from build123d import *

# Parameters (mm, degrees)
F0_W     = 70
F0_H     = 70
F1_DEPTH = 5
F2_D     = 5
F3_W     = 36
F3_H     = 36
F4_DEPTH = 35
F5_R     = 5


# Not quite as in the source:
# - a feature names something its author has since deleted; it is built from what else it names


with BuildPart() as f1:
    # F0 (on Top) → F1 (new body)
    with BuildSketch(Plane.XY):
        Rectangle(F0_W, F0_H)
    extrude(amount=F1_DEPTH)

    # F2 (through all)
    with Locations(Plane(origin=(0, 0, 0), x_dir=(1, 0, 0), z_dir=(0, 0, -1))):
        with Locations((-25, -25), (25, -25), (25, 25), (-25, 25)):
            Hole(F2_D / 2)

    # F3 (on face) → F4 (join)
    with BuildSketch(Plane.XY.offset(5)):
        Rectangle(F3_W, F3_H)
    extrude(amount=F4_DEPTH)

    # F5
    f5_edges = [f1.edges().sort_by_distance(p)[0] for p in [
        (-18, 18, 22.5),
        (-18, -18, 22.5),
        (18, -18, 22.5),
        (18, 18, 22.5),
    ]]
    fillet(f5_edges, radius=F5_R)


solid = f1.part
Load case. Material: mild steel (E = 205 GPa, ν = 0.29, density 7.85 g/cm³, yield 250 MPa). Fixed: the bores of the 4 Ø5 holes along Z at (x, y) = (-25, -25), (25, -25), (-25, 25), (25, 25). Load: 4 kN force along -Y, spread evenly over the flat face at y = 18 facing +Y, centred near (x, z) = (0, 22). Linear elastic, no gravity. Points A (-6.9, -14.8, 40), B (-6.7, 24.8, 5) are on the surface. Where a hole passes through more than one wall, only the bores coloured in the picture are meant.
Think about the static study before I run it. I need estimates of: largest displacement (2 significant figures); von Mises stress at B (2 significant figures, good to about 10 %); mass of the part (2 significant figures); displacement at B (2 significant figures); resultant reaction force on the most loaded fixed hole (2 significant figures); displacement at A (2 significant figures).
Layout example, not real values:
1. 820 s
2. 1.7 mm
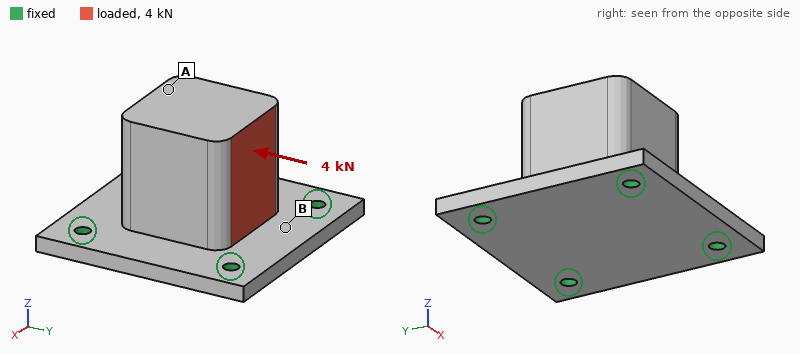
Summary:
1. 19 µm
2. 20 MPa
3. 540 g
4. 7.1 µm
5. 1.4 kN
6. 18 µm
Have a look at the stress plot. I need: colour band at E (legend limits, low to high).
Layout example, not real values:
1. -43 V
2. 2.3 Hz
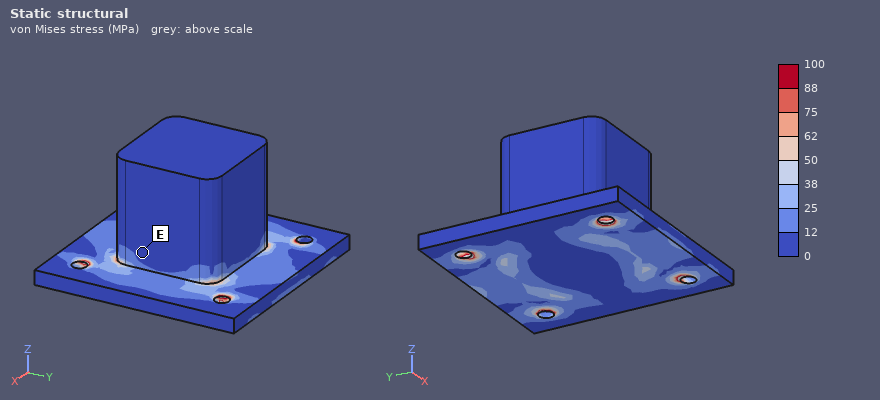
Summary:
1. 0 to 12 MPa
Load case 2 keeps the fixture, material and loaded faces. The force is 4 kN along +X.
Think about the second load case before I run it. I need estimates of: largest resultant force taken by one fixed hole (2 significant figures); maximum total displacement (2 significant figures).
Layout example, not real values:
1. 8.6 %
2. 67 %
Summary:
1. 1.7 kN
2. 20 µm
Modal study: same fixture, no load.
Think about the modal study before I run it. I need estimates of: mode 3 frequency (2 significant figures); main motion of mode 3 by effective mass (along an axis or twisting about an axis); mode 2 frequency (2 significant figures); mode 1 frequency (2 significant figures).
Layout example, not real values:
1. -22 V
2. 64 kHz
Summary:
1. 5000 Hz
2. along Z
3. 4500 Hz
4. 4500 Hz
